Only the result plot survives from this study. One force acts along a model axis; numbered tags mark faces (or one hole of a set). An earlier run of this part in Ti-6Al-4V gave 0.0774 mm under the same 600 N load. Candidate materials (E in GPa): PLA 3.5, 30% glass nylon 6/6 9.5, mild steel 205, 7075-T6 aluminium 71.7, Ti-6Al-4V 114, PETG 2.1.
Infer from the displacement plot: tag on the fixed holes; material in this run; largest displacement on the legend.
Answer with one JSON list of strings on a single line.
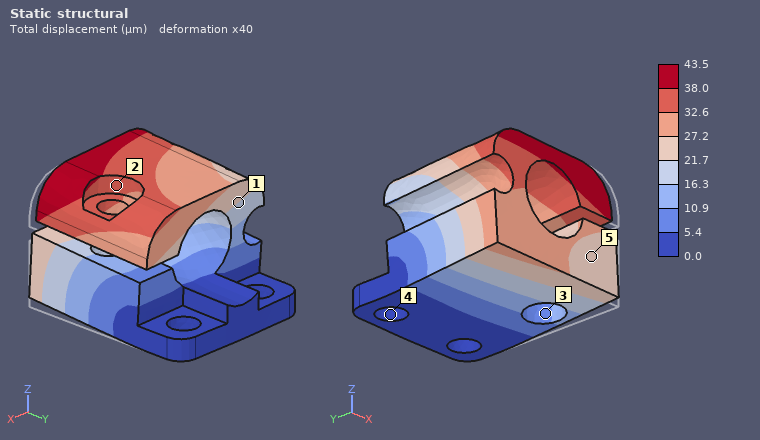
["4", "mild steel", "43.5 µm"]
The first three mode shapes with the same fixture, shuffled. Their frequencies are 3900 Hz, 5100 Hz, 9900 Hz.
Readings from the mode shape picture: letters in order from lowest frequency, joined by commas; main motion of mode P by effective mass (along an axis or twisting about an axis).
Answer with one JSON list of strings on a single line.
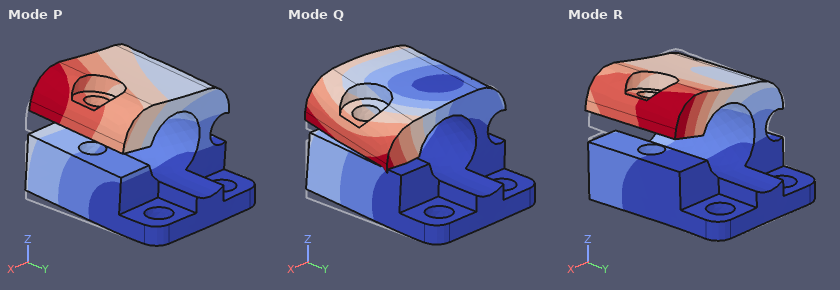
["P, R, Q", "along Z"]
